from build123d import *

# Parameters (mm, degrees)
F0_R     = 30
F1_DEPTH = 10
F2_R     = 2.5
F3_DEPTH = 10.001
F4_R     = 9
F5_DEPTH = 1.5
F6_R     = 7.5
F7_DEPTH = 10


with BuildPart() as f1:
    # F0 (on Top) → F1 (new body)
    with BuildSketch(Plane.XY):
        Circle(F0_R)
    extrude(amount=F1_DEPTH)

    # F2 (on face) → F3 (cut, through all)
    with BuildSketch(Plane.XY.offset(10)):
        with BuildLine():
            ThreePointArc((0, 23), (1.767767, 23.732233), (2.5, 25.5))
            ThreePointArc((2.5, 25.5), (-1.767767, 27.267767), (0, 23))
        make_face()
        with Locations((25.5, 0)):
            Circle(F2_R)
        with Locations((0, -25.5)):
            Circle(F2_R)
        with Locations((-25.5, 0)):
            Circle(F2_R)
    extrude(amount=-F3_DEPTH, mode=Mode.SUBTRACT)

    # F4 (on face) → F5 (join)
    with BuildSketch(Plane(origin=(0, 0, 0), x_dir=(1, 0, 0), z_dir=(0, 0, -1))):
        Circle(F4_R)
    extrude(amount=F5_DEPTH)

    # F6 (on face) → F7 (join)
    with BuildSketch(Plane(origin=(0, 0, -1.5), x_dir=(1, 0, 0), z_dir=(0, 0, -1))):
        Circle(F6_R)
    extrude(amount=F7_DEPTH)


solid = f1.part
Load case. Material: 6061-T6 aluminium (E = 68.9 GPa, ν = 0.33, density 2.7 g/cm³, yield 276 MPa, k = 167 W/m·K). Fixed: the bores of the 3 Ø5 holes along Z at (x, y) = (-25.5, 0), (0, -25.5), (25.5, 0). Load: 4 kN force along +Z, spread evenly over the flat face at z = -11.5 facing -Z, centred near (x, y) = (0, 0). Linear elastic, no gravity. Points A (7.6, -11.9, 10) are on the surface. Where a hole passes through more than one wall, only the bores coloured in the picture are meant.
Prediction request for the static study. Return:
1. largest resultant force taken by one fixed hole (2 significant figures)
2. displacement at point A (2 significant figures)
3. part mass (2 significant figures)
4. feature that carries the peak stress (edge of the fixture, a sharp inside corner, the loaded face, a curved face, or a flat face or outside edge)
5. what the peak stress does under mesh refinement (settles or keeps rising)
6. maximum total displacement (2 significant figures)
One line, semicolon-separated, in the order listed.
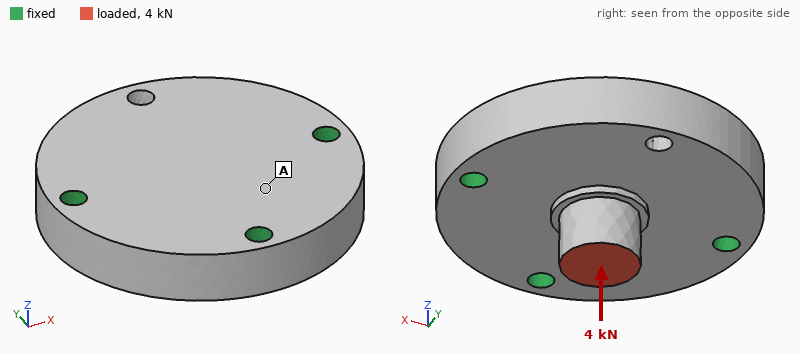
1.6 kN; 7.4 µm; 80 g; edge of the fixture; keeps rising; 27 µm
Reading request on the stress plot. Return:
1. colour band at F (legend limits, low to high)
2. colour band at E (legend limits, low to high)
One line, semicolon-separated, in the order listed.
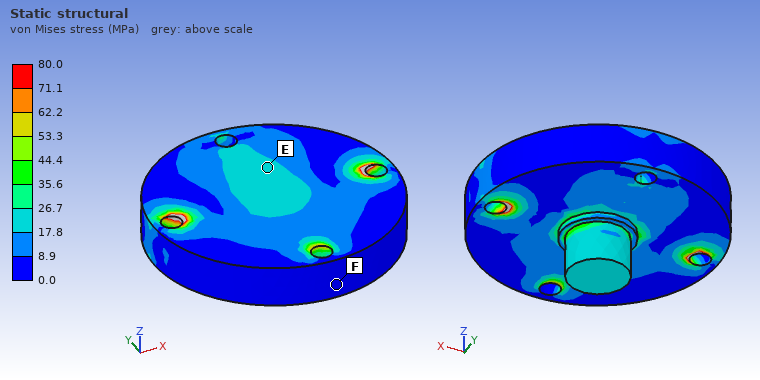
0.0 to 8.9 MPa; 17.8 to 26.7 MPa
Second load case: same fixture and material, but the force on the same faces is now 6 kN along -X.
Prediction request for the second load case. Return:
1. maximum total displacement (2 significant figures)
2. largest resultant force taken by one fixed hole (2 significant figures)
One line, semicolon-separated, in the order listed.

70 µm; 3.4 kN
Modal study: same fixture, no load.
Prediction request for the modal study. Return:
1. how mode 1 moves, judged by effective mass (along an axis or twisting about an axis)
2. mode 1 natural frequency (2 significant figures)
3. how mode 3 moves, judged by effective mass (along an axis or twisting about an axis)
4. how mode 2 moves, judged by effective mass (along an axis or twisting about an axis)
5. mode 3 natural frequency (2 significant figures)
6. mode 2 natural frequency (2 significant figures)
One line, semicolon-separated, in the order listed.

along Z; 8000 Hz; along Z; twisting about Y; 20 kHz; 19 kHz
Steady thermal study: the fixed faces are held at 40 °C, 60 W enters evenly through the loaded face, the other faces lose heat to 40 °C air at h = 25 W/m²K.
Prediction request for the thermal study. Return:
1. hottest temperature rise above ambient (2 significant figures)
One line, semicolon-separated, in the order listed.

37 K
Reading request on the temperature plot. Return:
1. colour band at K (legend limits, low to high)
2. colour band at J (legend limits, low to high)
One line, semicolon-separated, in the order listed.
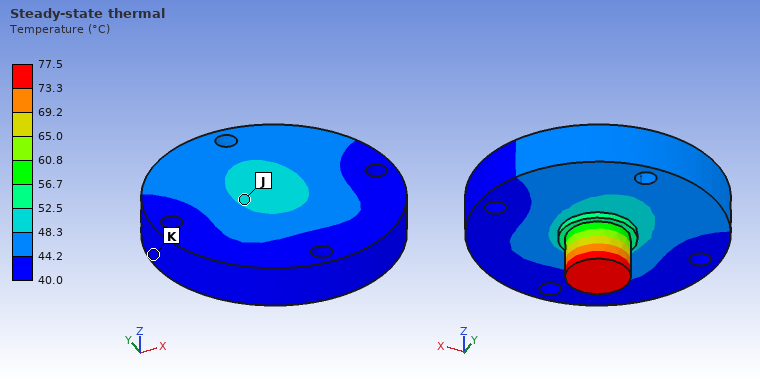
40.0 to 44.2 °C; 48.3 to 52.5 °C
